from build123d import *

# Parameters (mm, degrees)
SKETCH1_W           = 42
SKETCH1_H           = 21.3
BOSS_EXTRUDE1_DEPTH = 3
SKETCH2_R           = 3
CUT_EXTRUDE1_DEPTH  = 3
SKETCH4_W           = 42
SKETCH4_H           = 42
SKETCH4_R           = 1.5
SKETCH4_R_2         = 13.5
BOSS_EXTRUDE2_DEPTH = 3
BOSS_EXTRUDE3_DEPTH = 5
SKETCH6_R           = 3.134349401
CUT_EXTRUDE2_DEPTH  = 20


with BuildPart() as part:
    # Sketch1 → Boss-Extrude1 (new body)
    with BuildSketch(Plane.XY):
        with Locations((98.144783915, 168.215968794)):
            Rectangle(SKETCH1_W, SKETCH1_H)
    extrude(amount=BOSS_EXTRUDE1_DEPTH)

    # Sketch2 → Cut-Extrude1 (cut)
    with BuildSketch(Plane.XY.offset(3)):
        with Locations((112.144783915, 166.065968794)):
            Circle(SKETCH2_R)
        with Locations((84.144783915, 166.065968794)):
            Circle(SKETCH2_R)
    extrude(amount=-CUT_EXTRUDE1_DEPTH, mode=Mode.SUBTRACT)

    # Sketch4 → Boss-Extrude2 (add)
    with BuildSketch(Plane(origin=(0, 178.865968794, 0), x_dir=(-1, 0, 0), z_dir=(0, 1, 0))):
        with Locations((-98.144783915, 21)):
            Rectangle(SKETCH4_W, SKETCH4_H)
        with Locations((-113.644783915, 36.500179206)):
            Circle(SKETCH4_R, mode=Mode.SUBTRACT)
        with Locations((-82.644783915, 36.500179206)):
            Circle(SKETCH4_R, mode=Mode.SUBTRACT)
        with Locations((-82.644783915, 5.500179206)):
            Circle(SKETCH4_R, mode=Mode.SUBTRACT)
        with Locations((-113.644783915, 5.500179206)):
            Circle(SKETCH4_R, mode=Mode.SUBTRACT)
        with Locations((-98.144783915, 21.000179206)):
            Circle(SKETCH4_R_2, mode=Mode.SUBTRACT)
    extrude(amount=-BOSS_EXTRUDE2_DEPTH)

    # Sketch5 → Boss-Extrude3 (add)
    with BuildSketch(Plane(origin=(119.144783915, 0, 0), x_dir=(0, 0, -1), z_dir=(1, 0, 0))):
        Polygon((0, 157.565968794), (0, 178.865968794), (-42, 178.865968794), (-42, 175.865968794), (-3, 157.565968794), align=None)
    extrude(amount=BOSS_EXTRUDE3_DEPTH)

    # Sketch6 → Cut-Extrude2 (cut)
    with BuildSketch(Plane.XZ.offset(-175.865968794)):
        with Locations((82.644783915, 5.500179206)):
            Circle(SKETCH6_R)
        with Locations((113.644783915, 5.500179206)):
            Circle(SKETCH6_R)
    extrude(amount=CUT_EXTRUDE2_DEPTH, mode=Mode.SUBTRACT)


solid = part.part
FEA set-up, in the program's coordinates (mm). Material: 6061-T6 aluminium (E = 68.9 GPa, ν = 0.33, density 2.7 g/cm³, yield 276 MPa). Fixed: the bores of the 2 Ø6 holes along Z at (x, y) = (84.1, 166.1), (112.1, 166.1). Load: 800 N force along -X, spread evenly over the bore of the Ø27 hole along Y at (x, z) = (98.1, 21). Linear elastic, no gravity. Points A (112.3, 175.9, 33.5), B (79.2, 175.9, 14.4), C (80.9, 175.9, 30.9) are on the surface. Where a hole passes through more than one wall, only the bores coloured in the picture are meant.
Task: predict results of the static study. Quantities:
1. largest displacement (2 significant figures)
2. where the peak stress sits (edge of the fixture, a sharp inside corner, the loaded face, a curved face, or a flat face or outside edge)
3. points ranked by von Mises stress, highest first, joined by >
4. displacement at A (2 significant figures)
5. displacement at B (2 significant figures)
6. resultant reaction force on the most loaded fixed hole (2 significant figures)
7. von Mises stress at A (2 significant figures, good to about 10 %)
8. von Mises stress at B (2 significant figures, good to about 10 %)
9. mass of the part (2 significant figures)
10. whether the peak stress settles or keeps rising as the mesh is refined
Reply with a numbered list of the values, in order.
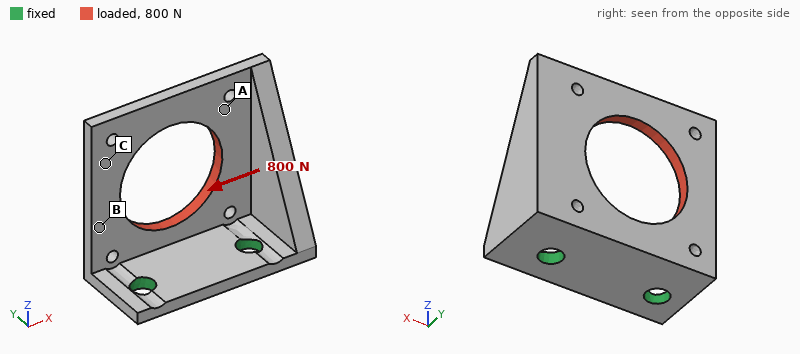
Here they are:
1. 0.19 mm
2. edge of the fixture
3. B > A > C
4. 0.14 mm
5. 0.080 mm
6. 670 N
7. 24 MPa
8. 46 MPa
9. 22 g
10. keeps rising
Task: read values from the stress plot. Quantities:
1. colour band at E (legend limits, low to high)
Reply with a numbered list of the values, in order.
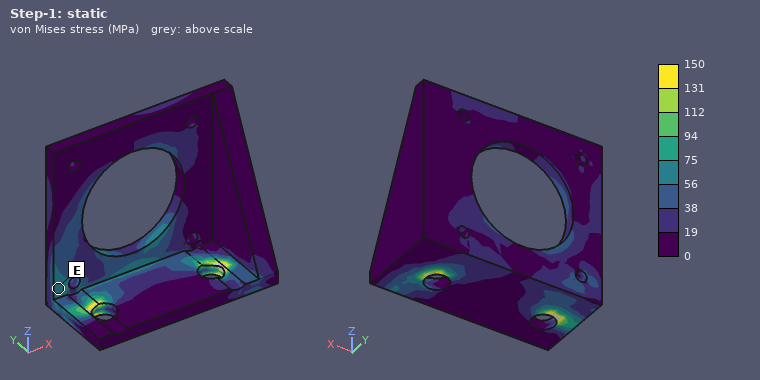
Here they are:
1. 56 to 75 MPa
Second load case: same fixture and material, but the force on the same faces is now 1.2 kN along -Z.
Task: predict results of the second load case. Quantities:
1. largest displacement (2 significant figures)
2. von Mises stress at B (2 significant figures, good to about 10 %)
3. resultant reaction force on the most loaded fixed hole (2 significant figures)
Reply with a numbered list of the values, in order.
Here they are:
1. 0.28 mm
2. 29 MPa
3. 610 N
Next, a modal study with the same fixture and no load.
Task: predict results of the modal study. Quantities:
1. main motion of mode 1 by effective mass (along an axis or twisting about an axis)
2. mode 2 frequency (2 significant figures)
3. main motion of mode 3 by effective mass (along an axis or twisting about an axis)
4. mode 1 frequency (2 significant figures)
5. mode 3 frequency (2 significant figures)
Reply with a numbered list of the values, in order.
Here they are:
1. along Y
2. 2700 Hz
3. along X
4. 1600 Hz
5. 4500 Hz
